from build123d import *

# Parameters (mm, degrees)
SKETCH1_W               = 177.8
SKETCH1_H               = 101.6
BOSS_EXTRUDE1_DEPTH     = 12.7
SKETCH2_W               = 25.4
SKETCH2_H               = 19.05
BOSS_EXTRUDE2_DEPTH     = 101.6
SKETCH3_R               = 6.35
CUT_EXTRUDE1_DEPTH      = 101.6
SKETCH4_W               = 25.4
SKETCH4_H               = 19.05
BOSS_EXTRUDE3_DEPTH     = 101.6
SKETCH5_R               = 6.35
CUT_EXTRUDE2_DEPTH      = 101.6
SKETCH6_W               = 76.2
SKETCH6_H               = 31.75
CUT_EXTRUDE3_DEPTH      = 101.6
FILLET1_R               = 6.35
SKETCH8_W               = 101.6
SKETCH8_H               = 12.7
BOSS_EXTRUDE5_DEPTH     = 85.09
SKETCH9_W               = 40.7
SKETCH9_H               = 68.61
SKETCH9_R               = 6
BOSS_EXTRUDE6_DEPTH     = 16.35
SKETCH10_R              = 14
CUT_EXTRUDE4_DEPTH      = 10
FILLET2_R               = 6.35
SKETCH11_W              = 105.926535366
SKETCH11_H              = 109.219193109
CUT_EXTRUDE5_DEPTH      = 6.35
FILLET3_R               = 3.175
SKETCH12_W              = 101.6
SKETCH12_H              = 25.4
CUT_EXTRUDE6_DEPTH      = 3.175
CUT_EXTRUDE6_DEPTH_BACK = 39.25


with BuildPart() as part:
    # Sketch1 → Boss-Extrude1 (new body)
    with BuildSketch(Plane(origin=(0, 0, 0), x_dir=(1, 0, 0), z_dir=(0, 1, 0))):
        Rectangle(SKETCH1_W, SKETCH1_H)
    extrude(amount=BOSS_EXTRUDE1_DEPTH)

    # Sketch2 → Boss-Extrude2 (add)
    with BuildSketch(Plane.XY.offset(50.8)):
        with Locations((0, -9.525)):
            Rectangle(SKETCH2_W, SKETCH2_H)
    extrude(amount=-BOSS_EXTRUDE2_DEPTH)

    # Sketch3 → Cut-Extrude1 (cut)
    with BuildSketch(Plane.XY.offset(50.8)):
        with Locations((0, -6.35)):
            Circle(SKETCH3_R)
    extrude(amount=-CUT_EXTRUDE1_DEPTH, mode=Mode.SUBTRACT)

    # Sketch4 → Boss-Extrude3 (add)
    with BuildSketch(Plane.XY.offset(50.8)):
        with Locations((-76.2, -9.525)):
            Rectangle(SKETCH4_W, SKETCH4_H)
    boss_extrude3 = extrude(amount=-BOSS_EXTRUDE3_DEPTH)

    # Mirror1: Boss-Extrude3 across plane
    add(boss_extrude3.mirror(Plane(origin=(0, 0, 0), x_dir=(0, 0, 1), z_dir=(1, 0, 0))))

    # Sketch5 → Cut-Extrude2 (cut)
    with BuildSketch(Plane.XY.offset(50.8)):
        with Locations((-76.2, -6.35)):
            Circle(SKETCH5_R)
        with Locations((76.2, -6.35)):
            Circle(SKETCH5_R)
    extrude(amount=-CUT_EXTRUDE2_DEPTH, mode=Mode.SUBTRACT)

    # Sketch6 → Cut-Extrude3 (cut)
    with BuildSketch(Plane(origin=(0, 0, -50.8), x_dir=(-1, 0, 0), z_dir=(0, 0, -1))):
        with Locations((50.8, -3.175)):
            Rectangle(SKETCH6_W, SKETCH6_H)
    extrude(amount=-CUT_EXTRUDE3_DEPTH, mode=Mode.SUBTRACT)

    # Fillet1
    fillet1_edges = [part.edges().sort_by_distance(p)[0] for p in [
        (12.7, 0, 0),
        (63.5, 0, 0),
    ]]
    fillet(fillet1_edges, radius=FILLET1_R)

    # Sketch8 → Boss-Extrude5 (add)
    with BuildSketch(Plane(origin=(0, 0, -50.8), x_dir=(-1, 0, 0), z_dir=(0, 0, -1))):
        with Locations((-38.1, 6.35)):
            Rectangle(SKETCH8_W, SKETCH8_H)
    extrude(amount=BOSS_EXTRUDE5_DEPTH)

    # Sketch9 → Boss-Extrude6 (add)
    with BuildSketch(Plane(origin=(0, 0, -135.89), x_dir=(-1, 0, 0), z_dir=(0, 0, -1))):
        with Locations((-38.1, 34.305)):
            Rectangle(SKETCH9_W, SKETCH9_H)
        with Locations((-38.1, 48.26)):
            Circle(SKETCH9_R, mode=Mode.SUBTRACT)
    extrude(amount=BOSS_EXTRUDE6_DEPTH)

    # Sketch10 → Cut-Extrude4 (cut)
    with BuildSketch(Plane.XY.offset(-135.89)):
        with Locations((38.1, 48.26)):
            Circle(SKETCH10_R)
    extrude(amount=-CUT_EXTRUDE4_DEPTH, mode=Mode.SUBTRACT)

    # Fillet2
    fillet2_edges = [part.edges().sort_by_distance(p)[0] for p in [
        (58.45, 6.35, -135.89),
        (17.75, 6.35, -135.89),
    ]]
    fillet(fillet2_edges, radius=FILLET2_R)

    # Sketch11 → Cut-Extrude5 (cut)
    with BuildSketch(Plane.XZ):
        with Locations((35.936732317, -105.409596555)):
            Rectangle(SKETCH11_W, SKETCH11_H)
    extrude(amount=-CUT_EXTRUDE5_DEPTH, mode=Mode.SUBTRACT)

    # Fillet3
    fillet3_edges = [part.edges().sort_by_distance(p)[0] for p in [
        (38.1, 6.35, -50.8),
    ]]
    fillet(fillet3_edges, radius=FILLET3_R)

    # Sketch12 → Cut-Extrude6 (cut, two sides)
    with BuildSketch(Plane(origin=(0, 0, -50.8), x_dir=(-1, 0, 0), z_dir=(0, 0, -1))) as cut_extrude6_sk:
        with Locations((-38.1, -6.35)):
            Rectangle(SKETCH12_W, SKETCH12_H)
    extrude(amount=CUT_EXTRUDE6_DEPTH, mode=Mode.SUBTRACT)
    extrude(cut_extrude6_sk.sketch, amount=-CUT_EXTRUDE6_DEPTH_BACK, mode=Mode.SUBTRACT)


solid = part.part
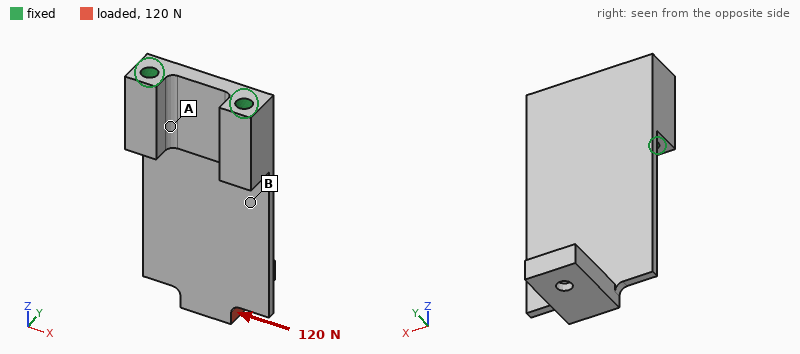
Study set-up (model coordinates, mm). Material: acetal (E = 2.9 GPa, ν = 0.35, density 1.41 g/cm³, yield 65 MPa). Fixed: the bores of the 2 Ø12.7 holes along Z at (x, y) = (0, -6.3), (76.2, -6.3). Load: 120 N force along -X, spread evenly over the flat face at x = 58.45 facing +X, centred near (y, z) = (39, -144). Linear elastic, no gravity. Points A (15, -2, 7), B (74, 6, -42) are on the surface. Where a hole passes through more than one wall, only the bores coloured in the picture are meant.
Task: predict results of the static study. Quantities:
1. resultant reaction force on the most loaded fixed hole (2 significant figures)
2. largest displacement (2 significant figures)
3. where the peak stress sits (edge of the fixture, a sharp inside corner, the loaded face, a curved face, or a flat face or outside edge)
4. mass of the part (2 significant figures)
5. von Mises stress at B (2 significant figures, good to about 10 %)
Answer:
230 N
2.8 mm
a curved face
340 g
3.7 MPa
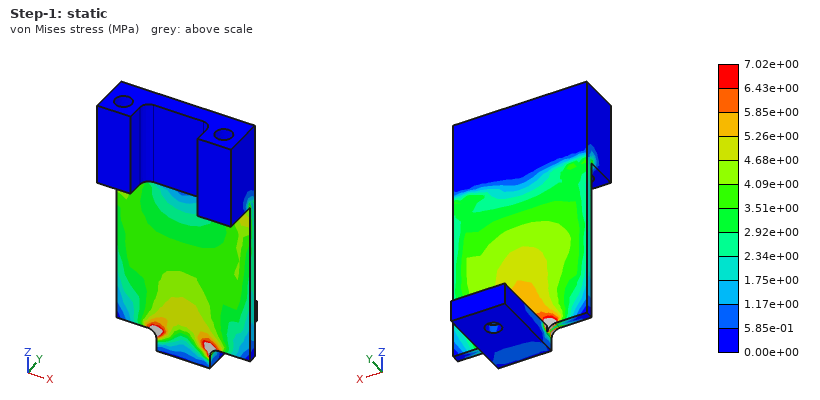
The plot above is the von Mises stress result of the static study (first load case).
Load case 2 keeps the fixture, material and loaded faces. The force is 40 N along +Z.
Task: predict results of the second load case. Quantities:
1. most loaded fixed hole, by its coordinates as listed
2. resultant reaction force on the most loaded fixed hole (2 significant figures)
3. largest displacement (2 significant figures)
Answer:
(76.2, -6.3)
30 N
2.5 mm
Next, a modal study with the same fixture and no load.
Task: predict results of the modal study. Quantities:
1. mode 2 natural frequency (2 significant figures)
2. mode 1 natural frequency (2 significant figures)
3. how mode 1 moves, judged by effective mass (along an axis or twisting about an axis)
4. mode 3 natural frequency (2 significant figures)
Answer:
160 Hz
50 Hz
along Y
230 Hz
